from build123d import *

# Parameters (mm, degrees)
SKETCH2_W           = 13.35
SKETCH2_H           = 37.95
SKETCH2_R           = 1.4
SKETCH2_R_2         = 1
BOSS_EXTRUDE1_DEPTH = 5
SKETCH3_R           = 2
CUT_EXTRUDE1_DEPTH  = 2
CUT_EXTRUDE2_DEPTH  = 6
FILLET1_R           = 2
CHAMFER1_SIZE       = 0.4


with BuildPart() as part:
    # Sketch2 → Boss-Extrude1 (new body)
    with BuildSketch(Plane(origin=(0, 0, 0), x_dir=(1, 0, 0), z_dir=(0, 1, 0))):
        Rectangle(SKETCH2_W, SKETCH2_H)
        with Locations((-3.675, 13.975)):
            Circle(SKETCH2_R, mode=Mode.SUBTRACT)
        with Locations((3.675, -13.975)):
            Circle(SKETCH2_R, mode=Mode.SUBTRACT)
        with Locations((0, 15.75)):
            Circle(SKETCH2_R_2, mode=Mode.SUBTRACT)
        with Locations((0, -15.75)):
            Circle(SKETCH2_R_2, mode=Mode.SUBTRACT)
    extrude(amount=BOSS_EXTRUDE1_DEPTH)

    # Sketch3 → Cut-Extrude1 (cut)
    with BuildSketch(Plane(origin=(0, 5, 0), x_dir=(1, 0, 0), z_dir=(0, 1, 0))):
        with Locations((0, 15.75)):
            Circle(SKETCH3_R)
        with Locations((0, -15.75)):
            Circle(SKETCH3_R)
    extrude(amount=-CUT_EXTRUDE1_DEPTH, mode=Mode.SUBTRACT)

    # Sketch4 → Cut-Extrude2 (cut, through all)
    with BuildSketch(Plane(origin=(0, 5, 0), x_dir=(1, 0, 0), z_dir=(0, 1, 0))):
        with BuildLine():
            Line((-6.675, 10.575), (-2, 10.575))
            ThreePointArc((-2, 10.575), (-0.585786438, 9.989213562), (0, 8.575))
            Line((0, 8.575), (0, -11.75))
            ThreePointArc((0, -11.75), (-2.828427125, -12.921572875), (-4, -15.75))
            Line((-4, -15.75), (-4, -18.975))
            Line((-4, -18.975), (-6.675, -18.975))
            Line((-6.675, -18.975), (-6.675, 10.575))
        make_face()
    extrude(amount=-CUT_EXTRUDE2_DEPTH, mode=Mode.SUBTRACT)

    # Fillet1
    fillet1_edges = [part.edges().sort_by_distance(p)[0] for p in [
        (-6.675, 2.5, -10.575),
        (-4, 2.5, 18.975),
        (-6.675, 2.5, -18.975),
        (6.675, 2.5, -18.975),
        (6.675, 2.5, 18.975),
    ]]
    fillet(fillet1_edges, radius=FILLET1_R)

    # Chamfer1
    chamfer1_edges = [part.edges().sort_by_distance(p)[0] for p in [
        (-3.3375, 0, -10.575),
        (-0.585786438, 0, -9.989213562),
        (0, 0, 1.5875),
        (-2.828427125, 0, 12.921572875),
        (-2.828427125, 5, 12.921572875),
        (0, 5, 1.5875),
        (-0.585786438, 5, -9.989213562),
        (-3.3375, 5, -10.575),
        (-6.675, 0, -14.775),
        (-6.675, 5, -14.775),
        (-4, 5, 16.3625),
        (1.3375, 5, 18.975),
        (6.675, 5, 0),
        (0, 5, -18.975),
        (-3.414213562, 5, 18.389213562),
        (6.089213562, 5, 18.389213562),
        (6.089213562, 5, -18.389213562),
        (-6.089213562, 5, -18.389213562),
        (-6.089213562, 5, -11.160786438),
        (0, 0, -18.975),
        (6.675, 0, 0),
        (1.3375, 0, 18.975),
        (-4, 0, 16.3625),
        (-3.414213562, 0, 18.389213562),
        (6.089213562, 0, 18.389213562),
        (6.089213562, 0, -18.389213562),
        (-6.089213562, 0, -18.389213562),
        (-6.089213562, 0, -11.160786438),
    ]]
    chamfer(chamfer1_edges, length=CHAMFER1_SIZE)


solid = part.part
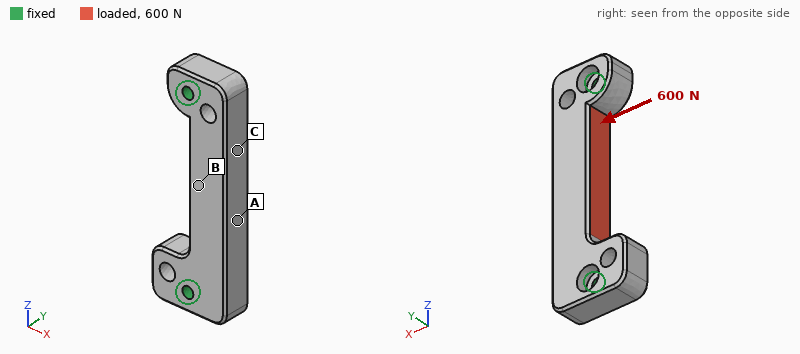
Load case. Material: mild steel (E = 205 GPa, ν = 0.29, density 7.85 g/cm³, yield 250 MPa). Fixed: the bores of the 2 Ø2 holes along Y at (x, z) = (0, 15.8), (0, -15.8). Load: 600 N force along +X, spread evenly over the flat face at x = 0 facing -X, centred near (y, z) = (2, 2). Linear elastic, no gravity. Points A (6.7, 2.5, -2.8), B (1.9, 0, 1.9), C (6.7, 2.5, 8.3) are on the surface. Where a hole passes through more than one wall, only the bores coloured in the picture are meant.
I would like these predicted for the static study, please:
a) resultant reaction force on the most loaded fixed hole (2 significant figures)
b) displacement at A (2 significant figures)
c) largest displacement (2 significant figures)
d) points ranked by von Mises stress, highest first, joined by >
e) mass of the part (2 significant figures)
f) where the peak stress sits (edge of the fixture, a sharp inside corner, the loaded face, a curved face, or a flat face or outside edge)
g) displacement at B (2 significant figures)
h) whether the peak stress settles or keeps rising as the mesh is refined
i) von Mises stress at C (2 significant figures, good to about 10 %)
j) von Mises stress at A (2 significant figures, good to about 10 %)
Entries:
450 N
4.9 µm
5.5 µm
A > C > B
12 g
edge of the fixture
4.9 µm
keeps rising
21 MPa
41 MPa
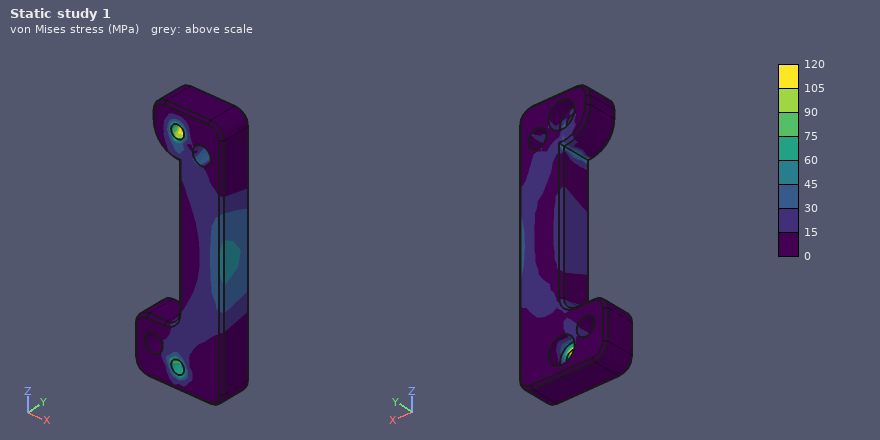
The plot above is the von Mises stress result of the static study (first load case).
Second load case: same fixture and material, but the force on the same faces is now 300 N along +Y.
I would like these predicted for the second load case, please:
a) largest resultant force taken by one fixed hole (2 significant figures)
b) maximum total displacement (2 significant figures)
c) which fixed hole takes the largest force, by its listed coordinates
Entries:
170 N
6.0 µm
(0, 15.8)
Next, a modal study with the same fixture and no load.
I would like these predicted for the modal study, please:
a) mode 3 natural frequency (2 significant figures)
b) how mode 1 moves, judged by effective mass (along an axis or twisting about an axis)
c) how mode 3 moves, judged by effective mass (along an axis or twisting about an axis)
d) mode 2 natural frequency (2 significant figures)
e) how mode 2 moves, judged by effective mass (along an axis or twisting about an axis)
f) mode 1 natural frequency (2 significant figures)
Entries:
32 kHz
along Y
twisting about Z
25 kHz
along X
16 kHz
